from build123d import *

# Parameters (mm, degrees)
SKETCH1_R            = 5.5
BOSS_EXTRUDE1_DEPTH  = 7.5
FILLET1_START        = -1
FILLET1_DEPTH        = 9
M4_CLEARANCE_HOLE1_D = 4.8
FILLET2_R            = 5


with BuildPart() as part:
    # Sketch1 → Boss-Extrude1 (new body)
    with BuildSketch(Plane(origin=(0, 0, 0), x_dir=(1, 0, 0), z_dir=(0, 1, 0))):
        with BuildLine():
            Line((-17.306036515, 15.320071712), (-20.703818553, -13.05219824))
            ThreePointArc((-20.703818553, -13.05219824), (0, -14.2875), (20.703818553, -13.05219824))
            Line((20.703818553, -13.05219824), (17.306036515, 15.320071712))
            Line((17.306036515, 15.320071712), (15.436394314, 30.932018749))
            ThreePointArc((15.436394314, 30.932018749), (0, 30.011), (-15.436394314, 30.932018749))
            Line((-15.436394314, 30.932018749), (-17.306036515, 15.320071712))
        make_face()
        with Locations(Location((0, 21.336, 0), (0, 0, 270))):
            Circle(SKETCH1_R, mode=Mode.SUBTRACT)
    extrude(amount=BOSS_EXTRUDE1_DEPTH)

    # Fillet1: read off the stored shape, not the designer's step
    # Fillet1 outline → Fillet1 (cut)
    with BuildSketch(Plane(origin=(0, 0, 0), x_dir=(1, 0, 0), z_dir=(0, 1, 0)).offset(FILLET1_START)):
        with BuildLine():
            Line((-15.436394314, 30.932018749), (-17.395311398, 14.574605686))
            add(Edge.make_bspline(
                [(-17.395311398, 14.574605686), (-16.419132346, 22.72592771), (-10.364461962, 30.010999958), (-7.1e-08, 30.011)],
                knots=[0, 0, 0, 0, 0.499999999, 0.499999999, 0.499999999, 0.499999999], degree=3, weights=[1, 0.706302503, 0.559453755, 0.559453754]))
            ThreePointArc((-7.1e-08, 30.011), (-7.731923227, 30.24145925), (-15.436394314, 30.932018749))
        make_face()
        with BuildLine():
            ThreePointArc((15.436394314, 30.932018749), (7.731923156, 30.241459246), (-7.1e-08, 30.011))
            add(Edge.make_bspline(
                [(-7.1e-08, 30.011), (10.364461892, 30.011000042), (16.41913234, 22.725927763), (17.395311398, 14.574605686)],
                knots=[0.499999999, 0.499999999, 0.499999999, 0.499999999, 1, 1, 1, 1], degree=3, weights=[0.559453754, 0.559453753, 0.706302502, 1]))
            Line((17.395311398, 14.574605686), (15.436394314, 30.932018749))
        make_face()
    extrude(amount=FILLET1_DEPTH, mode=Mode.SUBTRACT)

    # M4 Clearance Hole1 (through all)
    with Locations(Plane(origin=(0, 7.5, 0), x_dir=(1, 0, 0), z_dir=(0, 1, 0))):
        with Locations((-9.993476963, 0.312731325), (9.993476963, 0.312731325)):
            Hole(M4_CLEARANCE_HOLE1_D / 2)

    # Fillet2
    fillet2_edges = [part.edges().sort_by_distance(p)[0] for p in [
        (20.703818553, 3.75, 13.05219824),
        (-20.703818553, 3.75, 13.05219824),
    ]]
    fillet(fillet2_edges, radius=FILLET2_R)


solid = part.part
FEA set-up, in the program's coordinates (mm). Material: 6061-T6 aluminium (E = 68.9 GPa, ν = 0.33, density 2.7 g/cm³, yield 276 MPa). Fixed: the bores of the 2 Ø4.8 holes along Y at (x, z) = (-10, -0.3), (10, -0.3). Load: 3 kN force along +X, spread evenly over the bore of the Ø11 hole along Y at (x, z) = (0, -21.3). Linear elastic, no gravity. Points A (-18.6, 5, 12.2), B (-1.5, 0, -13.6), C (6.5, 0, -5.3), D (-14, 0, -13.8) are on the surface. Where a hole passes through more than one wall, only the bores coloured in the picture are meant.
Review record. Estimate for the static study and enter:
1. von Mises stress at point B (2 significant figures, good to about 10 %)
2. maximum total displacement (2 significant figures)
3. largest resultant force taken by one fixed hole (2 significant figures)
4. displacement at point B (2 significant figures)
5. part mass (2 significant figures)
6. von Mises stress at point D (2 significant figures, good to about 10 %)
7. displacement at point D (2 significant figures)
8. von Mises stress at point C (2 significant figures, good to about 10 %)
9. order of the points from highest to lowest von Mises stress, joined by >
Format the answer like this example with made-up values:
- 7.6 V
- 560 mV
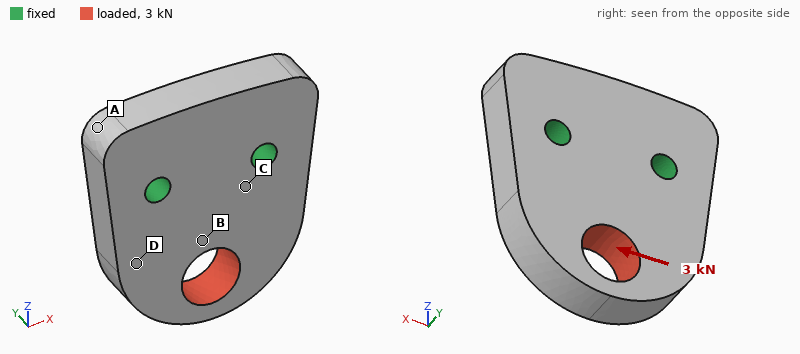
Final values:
- 47 MPa
- 29 µm
- 3.0 kN
- 9.8 µm
- 27 g
- 19 MPa
- 12 µm
- 31 MPa
- B > C > D > A
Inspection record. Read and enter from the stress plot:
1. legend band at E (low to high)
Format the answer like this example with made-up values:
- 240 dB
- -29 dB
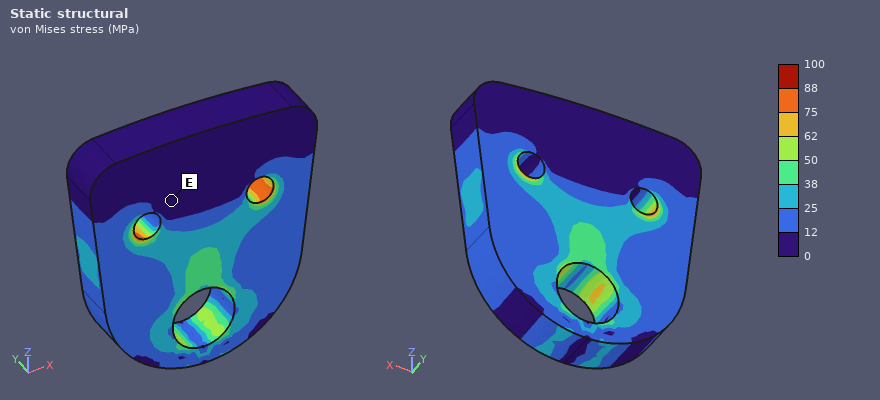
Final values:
- 0 to 12 MPa
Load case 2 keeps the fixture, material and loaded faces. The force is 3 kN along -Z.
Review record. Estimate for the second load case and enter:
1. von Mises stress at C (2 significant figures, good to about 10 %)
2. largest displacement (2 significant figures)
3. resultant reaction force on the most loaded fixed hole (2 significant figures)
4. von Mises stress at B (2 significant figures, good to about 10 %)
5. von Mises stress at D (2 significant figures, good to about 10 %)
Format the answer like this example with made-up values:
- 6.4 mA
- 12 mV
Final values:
- 14 MPa
- 12 µm
- 1.5 kN
- 13 MPa
- 9.1 MPa
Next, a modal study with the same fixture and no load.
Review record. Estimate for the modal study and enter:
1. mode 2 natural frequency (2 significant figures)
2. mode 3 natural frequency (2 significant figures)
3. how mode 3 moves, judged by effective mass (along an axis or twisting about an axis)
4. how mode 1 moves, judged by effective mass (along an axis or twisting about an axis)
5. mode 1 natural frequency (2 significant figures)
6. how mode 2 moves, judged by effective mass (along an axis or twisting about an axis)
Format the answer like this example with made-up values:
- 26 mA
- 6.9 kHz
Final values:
- 17 kHz
- 22 kHz
- along X
- along Y
- 9200 Hz
- twisting about Z
